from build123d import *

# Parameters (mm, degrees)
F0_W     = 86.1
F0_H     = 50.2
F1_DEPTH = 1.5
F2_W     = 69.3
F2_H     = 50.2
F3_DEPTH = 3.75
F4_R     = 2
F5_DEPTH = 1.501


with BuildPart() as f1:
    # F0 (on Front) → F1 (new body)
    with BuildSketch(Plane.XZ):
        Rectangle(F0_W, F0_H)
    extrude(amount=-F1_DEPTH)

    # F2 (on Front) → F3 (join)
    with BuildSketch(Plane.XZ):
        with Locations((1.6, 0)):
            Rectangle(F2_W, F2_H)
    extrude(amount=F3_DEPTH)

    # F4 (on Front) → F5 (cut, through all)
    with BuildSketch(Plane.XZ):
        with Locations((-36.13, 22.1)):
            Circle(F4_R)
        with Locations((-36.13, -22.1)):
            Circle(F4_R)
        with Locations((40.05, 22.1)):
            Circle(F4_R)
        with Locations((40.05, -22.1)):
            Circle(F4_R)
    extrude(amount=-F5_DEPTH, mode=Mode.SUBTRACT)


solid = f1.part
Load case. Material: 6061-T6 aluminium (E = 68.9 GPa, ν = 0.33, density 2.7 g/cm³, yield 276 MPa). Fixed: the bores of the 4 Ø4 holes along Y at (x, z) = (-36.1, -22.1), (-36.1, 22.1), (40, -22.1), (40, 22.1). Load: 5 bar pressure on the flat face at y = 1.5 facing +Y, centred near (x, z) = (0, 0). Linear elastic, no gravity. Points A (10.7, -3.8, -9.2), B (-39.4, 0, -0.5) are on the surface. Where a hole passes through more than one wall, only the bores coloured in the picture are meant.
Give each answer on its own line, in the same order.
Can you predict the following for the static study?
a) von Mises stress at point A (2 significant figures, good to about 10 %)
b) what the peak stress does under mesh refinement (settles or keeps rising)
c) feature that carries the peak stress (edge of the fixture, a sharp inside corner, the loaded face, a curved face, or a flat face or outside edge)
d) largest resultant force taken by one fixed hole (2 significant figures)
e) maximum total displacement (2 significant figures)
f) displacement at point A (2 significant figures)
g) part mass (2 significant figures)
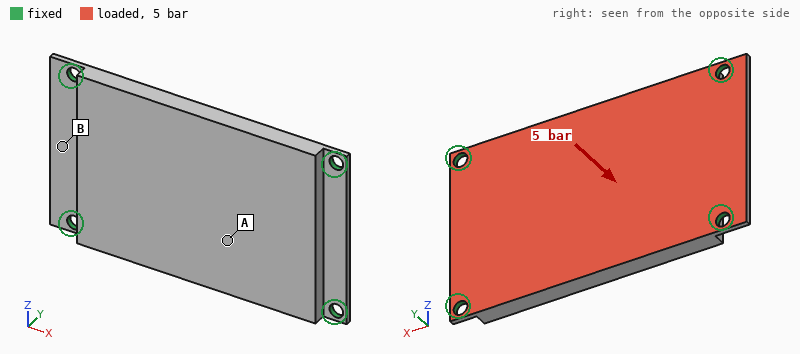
44 MPa
keeps rising
edge of the fixture
1.3 kN
0.14 mm
0.13 mm
53 g
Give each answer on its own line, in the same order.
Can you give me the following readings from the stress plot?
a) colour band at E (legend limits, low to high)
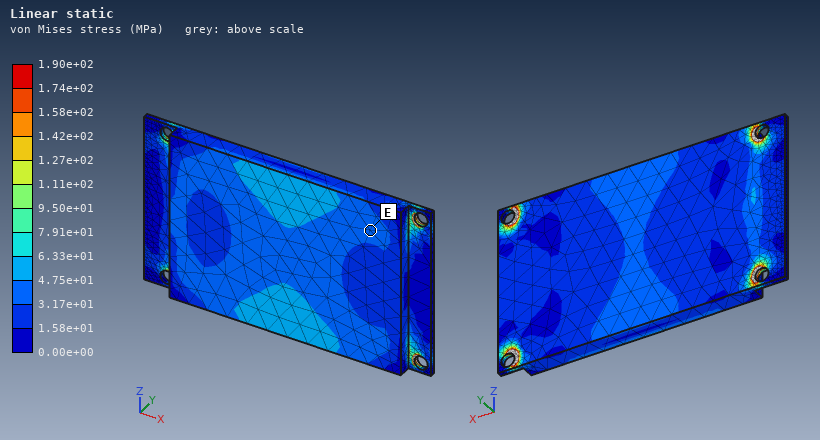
3.17e+01 to 4.75e+01 MPa
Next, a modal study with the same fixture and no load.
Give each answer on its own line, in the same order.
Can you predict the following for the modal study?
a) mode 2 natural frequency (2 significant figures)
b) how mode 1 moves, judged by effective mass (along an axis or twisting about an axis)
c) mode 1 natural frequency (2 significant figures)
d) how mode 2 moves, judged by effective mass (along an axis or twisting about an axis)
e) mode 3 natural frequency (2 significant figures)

5000 Hz
along Y
2800 Hz
twisting about X
6800 Hz
